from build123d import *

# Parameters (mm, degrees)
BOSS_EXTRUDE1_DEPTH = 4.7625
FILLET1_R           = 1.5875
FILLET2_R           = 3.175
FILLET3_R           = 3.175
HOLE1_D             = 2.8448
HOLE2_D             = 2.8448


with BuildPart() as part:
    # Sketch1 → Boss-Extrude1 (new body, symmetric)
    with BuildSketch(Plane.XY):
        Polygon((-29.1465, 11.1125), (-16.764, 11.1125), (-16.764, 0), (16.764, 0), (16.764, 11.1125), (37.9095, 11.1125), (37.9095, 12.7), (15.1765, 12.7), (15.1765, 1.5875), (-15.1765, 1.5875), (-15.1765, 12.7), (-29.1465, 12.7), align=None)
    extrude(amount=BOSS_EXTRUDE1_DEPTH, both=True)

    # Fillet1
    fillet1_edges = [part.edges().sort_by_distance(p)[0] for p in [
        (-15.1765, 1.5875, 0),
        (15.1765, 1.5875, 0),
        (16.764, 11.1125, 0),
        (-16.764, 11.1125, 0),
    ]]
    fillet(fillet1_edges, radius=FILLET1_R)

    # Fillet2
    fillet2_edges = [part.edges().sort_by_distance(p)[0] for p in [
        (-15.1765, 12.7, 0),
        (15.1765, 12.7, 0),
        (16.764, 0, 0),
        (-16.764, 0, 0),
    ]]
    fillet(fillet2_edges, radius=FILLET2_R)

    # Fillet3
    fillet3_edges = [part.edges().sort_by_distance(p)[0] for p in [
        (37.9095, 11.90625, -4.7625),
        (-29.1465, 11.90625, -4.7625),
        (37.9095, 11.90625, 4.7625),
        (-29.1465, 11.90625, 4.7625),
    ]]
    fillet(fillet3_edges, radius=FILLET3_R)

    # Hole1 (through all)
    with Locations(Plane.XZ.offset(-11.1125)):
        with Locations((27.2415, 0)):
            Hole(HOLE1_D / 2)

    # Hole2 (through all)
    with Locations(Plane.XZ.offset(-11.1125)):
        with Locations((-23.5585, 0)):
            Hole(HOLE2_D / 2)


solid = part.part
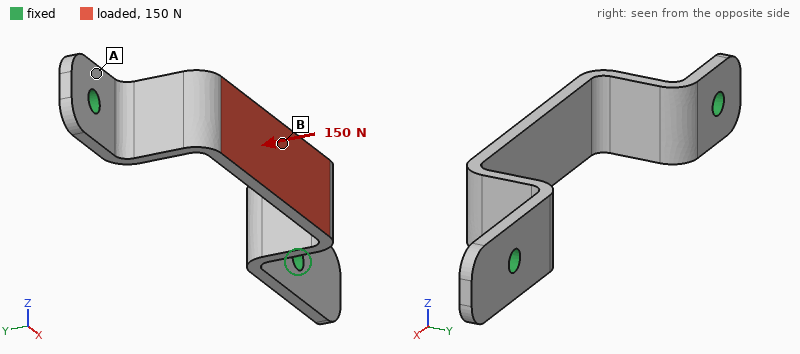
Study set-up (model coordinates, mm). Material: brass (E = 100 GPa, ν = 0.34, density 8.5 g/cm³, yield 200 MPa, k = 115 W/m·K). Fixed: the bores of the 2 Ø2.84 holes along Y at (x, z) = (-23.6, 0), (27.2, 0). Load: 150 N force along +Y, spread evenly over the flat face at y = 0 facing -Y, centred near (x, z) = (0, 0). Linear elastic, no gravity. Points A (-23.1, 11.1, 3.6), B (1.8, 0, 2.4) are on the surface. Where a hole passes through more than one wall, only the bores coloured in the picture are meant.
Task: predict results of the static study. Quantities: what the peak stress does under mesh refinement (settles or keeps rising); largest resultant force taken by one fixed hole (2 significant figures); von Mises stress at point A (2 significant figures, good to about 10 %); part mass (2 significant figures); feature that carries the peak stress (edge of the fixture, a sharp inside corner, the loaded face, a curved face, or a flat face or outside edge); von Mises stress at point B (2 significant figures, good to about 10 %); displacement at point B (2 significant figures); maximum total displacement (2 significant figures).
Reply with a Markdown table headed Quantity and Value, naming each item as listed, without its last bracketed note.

| Quantity | Value |
|---|---|
| what the peak stress does under mesh refinement | keeps rising |
| largest resultant force taken by one fixed hole | 100 N |
| von Mises stress at point A | 17 MPa |
| part mass | 11 g |
| feature that carries the peak stress | edge of the fixture |
| von Mises stress at point B | 66 MPa |
| displacement at point B | 74 µm |
| maximum total displacement | 76 µm |
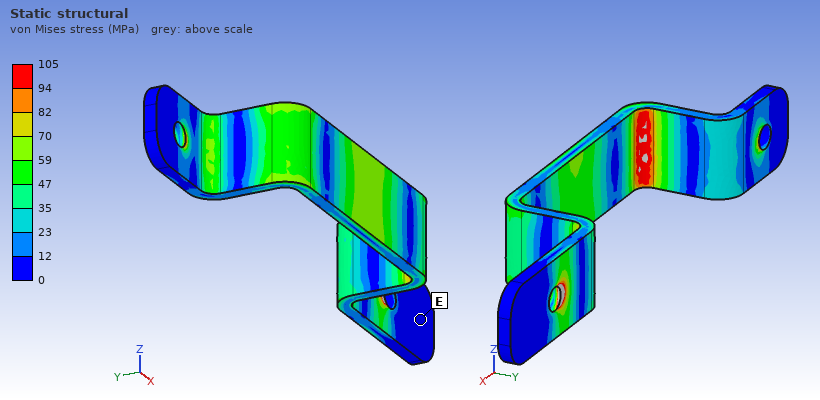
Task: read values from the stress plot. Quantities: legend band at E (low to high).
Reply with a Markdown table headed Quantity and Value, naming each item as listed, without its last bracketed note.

| Quantity | Value |
|---|---|
| legend band at E | 0 to 12 MPa |
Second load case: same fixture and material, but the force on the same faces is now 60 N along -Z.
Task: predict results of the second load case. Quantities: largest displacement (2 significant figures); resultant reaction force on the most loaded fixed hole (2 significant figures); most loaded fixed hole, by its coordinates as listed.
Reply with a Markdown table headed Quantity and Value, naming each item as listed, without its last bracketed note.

| Quantity | Value |
|---|---|
| largest displacement | 79 µm |
| resultant reaction force on the most loaded fixed hole | 33 N |
| most loaded fixed hole, by its coordinates as listed | (-23.6, 0) |
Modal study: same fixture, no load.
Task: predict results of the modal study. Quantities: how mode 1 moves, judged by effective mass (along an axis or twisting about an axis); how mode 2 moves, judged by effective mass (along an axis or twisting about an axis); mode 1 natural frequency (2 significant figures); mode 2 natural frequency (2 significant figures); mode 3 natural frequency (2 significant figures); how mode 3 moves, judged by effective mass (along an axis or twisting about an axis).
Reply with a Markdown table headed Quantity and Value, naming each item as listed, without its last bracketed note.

| Quantity | Value |
|---|---|
| how mode 1 moves, judged by effective mass | along Z |
| how mode 2 moves, judged by effective mass | along X |
| mode 1 natural frequency | 2200 Hz |
| mode 2 natural frequency | 2800 Hz |
| mode 3 natural frequency | 4000 Hz |
| how mode 3 moves, judged by effective mass | along Y |
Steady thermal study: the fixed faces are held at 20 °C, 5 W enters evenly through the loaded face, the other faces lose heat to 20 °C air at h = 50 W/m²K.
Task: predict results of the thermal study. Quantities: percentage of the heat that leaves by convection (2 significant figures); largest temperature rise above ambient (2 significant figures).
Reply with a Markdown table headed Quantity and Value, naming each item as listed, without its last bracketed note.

| Quantity | Value |
|---|---|
| percentage of the heat that leaves by convection | 21 % |
| largest temperature rise above ambient | 33 K |
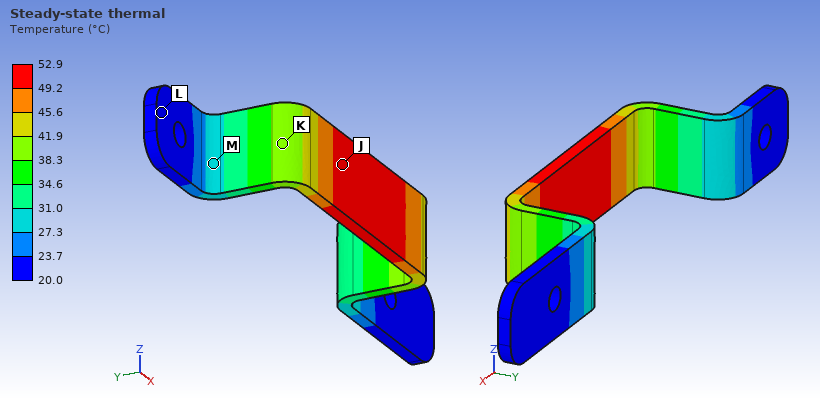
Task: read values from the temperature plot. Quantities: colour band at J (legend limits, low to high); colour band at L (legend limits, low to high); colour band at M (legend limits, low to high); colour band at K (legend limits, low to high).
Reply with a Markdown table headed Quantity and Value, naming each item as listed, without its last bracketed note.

| Quantity | Value |
|---|---|
| colour band at J | 49.2 to 52.9 °C |
| colour band at L | 20.0 to 23.7 °C |
| colour band at M | 27.3 to 31.0 °C |
| colour band at K | 38.3 to 41.9 °C |
